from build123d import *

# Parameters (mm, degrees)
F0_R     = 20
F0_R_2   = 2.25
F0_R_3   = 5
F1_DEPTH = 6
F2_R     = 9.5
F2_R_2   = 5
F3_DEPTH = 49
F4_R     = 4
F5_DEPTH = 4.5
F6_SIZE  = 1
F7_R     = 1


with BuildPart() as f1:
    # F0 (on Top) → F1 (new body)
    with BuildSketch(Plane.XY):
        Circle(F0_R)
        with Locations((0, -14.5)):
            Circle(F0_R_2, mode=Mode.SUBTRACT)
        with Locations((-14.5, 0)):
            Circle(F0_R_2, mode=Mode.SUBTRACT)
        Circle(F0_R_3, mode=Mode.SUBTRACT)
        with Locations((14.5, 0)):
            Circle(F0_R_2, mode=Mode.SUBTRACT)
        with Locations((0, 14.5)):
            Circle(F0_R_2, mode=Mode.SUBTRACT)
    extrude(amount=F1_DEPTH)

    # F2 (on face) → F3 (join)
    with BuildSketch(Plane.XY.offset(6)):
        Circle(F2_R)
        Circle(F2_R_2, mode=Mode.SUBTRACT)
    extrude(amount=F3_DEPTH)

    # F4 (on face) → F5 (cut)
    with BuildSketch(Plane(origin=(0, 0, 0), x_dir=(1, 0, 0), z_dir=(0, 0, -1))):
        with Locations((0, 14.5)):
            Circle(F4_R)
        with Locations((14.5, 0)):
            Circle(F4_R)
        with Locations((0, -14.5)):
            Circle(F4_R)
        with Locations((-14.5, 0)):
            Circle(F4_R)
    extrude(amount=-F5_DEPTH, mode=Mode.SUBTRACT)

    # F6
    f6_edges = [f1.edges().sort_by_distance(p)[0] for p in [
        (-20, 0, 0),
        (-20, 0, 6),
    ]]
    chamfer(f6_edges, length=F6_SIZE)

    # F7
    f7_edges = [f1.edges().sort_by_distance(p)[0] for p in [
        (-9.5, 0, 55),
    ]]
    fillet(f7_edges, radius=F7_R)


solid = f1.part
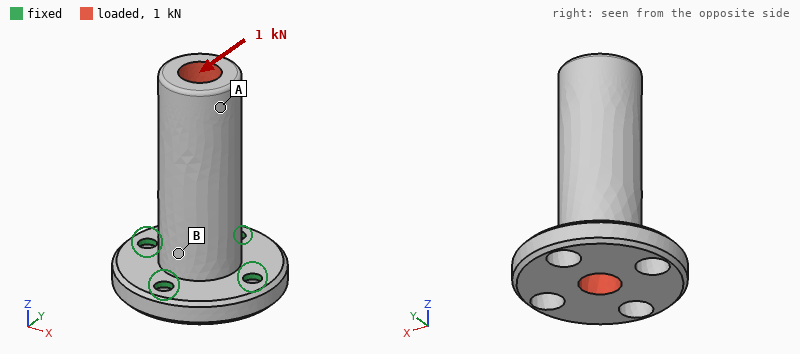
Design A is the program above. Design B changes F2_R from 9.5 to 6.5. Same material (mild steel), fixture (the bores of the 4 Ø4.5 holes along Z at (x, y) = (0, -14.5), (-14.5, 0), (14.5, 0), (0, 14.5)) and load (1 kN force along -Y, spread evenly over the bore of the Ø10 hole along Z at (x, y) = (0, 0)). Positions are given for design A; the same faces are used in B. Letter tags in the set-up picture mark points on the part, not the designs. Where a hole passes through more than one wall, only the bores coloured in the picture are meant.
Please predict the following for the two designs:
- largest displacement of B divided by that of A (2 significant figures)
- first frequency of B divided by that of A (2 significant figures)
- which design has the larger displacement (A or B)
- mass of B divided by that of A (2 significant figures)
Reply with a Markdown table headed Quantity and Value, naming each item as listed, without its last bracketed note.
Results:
| Quantity | Value |
|---|---|
| largest displacement of B divided by that of A | 4.2 |
| first frequency of B divided by that of A | 0.95 |
| which design has the larger displacement | B |
| mass of B divided by that of A | 0.54 |
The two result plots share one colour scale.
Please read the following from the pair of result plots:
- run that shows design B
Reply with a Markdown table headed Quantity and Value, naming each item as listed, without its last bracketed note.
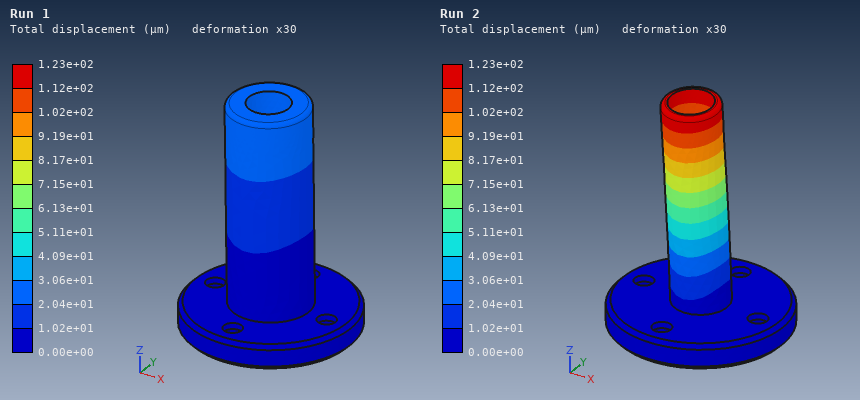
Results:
| Quantity | Value |
|---|---|
| run that shows design B | Run 2 |
